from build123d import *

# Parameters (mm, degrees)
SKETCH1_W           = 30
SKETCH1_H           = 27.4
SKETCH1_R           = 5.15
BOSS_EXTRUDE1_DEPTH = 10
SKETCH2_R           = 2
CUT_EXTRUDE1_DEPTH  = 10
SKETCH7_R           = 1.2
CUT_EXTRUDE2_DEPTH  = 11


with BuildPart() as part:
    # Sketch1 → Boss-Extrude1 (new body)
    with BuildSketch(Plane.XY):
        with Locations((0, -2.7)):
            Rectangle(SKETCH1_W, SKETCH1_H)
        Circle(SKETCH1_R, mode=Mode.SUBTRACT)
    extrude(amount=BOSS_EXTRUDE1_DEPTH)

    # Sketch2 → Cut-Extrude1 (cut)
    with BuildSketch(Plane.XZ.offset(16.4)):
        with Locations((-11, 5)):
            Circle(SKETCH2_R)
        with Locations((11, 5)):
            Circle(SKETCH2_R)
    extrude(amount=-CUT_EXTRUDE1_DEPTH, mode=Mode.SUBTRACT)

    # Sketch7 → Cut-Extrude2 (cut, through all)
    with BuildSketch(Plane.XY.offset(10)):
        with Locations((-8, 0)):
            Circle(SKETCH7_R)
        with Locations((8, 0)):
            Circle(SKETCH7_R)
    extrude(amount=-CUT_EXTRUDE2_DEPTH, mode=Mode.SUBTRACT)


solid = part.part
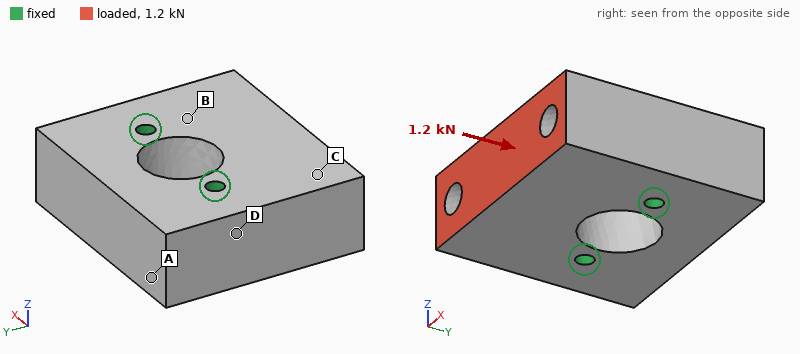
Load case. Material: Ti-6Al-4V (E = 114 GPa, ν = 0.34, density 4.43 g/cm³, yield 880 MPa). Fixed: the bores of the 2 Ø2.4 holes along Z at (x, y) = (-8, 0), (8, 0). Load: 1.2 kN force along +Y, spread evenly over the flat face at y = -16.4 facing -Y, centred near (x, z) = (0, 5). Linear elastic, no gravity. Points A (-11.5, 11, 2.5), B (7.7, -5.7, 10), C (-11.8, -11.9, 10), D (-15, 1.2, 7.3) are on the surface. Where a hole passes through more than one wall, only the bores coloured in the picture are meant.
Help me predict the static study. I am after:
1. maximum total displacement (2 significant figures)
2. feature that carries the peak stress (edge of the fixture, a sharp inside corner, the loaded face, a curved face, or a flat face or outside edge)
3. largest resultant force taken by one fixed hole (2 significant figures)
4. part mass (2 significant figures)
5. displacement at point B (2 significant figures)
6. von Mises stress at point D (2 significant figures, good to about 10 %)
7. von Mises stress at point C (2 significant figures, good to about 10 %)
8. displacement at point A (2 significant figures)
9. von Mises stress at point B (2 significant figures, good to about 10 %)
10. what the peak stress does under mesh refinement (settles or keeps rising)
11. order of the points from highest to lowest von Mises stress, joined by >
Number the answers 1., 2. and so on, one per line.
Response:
1. 0.90 µm
2. edge of the fixture
3. 610 N
4. 31 g
5. 0.36 µm
6. 2.3 MPa
7. 4.5 MPa
8. 0.19 µm
9. 6.7 MPa
10. keeps rising
11. B > C > D > A
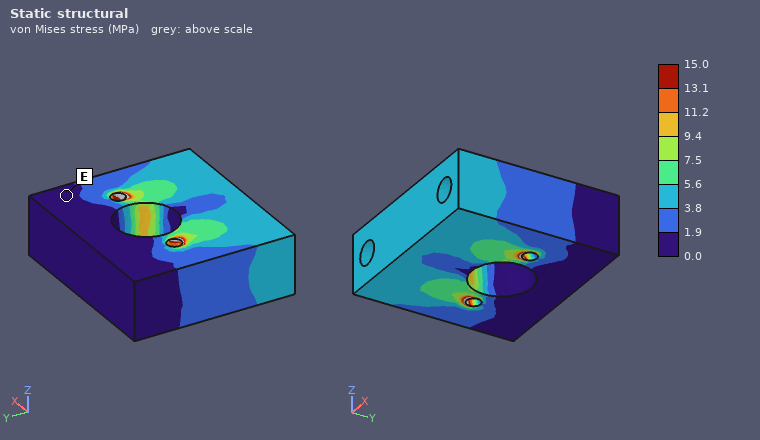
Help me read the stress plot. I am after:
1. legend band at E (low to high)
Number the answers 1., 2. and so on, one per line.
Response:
1. 0.0 to 1.9 MPa
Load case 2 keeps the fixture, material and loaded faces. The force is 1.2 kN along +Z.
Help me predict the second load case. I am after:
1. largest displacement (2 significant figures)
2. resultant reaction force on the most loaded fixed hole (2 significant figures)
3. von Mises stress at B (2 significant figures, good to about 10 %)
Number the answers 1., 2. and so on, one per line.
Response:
1. 14 µm
2. 600 N
3. 39 MPa
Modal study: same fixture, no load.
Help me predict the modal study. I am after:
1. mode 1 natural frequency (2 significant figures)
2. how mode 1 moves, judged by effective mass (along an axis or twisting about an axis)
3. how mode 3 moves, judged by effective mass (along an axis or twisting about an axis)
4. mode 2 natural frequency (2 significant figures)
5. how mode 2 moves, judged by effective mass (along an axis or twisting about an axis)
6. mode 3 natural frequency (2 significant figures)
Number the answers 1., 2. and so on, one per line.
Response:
1. 19 kHz
2. along Z
3. twisting about Y
4. 27 kHz
5. along X
6. 30 kHz
